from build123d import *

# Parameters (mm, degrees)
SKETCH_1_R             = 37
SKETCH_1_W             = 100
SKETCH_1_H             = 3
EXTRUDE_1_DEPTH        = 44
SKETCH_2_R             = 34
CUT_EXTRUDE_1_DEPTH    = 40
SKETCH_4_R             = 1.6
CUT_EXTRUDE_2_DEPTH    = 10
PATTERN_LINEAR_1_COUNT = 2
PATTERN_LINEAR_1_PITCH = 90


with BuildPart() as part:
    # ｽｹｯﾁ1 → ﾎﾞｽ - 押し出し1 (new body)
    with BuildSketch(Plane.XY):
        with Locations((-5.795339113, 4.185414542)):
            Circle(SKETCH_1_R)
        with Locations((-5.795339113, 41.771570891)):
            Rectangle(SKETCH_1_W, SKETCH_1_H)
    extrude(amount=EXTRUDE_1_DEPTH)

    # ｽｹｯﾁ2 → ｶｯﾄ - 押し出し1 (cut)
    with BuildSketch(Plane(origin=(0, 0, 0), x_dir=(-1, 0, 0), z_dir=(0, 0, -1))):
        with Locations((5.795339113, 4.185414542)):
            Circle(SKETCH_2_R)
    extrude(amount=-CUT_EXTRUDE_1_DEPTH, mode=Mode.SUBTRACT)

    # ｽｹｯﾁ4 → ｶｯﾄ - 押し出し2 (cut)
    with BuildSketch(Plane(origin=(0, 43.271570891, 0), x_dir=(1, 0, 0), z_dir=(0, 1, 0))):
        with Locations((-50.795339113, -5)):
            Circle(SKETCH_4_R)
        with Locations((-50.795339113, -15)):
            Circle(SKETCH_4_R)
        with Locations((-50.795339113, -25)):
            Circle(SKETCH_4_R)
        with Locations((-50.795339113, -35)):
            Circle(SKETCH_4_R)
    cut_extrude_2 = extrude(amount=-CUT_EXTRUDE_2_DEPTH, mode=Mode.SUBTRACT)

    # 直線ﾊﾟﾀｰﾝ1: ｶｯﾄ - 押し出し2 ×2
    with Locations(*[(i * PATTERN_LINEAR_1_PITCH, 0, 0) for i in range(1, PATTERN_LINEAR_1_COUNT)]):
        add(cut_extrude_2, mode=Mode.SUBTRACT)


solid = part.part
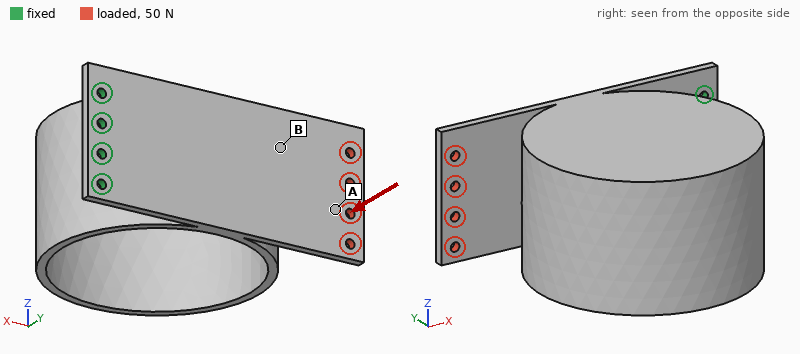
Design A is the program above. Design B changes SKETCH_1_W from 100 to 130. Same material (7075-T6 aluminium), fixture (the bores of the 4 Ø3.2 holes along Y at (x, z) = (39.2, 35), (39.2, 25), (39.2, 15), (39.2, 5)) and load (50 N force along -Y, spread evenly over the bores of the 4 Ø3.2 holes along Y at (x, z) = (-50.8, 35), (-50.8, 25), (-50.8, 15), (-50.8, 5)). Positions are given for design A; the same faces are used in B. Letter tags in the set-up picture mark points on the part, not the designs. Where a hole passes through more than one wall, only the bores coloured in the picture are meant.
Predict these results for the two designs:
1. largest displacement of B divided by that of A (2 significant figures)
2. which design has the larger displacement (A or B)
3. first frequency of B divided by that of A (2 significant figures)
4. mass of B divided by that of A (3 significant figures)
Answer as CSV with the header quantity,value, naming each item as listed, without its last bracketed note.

quantity,value
largest displacement of B divided by that of A,1.2
which design has the larger displacement,B
first frequency of B divided by that of A,0.96
mass of B divided by that of A,1.07
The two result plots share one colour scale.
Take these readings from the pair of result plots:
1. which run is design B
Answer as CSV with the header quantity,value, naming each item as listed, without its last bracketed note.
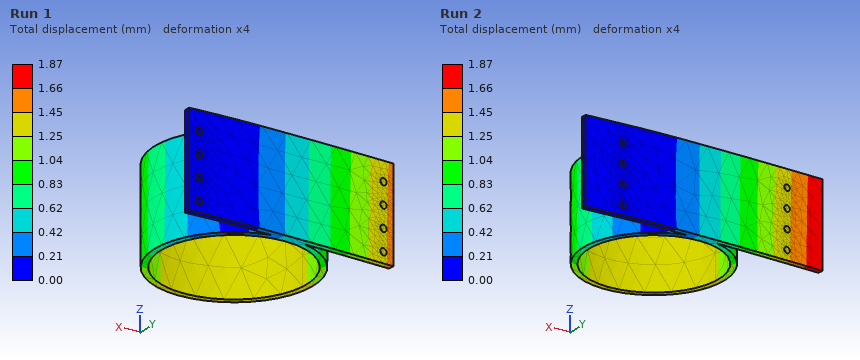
quantity,value
which run is design B,Run 2
